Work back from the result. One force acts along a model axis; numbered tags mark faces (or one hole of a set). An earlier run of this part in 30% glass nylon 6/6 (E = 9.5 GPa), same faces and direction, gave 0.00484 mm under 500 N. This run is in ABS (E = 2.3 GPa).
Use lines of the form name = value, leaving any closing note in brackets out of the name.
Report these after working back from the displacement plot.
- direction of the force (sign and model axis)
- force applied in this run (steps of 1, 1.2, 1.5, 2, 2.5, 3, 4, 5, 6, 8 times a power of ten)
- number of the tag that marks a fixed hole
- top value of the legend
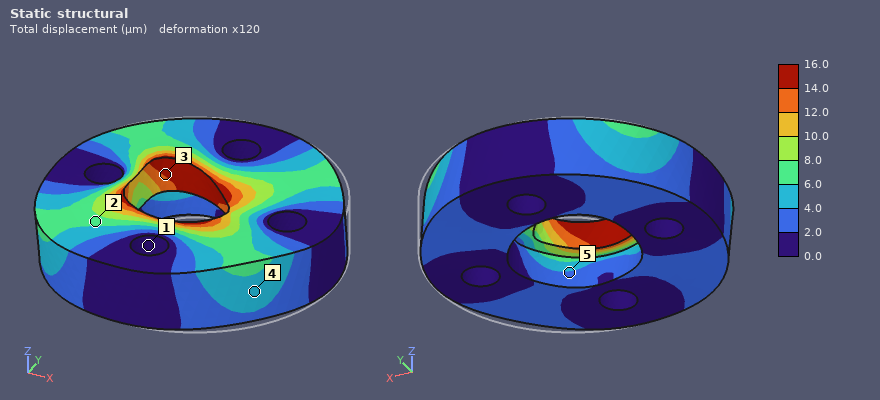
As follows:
direction of the force = -X
force applied in this run = 400 N
number of the tag that marks a fixed hole = 1
top value of the legend = 16.0 µm
